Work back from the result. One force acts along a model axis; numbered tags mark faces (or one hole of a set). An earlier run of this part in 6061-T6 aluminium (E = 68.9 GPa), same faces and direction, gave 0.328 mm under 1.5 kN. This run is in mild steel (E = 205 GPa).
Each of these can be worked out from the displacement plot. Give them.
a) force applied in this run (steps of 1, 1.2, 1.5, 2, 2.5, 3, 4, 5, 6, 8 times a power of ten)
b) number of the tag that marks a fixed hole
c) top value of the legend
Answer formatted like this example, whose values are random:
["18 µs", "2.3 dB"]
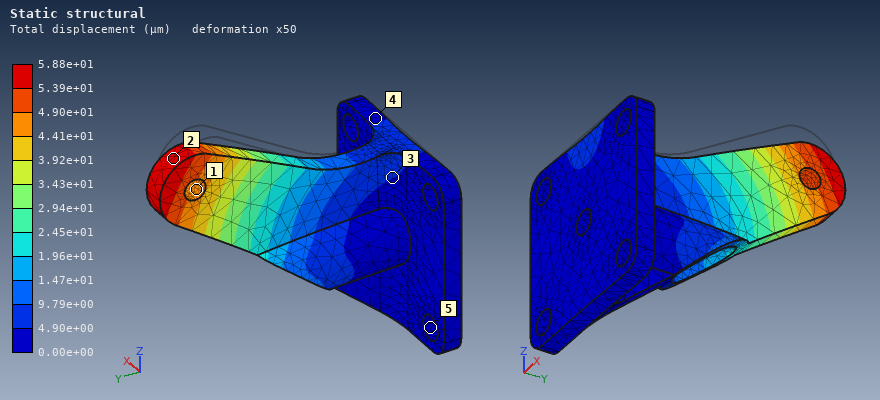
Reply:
["800 N", "5", "5.88e+01 µm"]
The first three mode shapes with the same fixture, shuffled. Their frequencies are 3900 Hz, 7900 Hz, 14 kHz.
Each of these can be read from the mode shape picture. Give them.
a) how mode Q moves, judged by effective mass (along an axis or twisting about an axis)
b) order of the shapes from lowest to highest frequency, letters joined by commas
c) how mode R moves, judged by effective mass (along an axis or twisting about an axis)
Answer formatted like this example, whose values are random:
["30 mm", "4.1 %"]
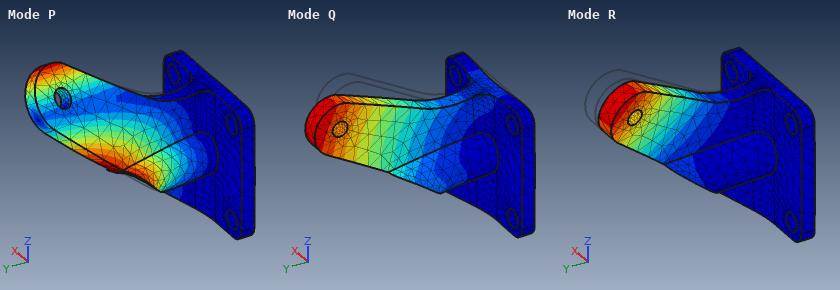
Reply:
["along Z", "R, Q, P", "along X"]
